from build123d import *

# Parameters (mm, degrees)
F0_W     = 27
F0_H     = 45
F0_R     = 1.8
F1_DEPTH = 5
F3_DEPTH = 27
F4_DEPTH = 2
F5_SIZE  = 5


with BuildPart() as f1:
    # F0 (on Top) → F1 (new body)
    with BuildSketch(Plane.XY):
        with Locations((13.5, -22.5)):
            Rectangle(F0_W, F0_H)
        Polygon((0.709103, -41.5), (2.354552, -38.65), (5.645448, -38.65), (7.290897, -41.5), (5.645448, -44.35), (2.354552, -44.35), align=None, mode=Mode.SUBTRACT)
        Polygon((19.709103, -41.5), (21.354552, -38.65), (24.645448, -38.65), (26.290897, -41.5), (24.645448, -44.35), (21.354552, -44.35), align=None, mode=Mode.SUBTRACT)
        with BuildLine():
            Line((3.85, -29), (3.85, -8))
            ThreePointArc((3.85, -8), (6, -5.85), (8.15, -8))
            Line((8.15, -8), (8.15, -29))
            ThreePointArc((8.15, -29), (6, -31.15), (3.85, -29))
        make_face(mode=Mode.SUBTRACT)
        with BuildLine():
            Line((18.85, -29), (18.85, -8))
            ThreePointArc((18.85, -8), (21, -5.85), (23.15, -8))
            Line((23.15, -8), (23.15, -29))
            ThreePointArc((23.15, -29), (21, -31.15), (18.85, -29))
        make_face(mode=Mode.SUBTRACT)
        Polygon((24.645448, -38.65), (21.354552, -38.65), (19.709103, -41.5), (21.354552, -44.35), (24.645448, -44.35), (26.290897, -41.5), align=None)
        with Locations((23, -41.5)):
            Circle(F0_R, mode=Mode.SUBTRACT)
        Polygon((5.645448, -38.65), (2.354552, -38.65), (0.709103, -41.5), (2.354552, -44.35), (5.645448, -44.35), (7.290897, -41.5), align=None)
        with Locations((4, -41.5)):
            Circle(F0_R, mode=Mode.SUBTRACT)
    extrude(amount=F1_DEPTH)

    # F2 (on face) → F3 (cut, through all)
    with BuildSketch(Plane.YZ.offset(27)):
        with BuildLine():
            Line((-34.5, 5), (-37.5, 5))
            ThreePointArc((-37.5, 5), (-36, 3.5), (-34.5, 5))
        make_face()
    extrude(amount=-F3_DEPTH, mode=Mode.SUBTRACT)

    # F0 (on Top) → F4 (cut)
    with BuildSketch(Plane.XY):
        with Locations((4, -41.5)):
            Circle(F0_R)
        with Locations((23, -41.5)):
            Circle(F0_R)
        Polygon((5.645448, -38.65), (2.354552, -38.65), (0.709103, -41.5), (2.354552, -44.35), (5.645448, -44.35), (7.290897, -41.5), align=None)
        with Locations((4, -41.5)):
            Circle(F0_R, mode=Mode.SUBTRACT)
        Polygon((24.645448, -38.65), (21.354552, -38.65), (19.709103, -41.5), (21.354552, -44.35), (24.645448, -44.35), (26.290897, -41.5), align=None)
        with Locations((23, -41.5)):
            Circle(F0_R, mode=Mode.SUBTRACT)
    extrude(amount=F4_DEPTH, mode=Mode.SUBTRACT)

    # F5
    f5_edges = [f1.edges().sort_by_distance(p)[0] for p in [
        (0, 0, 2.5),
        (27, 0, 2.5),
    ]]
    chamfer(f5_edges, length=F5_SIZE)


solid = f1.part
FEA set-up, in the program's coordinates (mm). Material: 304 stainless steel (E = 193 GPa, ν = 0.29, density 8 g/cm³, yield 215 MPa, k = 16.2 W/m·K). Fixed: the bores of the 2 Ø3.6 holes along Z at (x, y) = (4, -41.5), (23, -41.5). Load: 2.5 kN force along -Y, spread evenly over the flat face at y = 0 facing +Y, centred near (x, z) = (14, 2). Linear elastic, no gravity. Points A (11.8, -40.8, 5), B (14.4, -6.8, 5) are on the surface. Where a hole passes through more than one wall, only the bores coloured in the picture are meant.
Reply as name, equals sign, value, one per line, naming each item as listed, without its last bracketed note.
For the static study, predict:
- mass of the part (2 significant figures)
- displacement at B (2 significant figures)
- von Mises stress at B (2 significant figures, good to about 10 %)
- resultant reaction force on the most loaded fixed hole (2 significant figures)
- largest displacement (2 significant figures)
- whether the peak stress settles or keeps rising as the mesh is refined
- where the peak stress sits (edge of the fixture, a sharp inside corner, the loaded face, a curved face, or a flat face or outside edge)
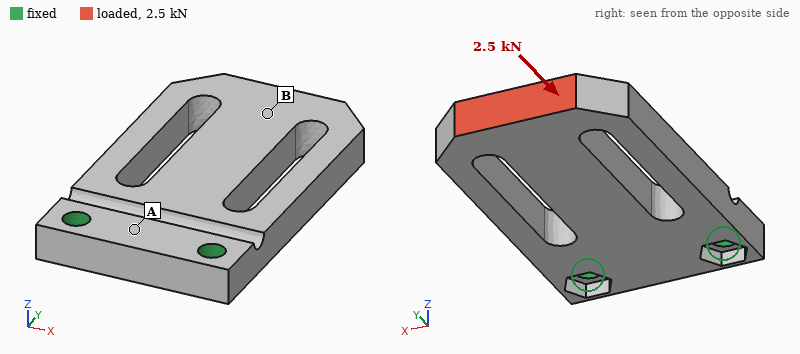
mass of the part = 37 g
displacement at B = 7.7 µm
von Mises stress at B = 40 MPa
resultant reaction force on the most loaded fixed hole = 1.3 kN
largest displacement = 9.4 µm
whether the peak stress settles or keeps rising as the mesh is refined = keeps rising
where the peak stress sits = edge of the fixture
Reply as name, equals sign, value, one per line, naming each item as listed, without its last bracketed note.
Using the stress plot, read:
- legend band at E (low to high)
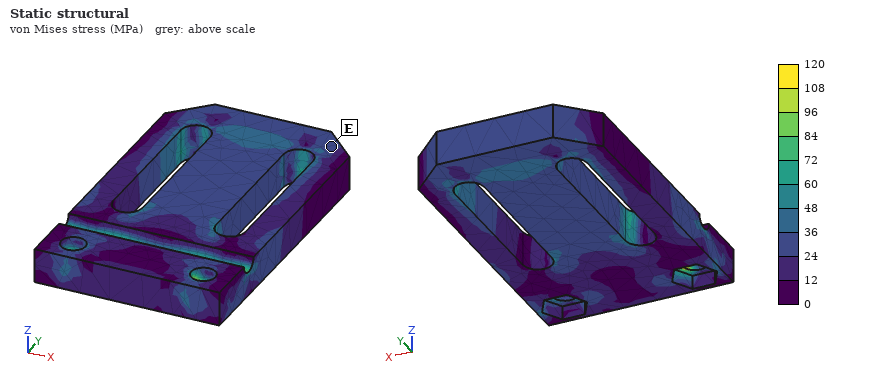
legend band at E = 24 to 36 MPa
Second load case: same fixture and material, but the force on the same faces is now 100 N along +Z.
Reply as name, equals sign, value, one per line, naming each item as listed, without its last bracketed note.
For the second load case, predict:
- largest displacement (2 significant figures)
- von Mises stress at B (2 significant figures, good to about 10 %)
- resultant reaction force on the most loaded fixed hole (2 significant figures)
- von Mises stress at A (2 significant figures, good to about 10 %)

largest displacement = 90 µm
von Mises stress at B = 11 MPa
resultant reaction force on the most loaded fixed hole = 53 N
von Mises stress at A = 18 MPa
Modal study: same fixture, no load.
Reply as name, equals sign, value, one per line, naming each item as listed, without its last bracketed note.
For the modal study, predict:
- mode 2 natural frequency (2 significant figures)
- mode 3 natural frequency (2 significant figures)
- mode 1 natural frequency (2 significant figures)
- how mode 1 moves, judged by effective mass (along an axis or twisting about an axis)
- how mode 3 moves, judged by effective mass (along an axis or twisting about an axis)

mode 2 natural frequency = 6300 Hz
mode 3 natural frequency = 6800 Hz
mode 1 natural frequency = 1800 Hz
how mode 1 moves, judged by effective mass = along Z
how mode 3 moves, judged by effective mass = along X
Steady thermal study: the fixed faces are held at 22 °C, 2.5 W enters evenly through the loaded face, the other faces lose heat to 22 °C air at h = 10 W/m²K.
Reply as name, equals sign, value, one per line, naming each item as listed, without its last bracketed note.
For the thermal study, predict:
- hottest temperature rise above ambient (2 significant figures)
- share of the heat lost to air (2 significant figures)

hottest temperature rise above ambient = 57 K
share of the heat lost to air = 29 %
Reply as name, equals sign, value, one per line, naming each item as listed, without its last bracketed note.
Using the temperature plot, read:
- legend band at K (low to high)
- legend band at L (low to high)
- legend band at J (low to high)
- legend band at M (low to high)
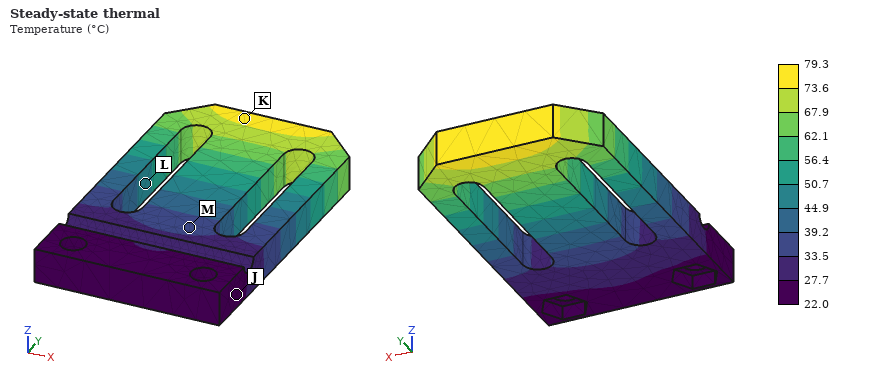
legend band at K = 73.6 to 79.3 °C
legend band at L = 44.9 to 50.7 °C
legend band at J = 22.0 to 27.7 °C
legend band at M = 33.5 to 39.2 °C
